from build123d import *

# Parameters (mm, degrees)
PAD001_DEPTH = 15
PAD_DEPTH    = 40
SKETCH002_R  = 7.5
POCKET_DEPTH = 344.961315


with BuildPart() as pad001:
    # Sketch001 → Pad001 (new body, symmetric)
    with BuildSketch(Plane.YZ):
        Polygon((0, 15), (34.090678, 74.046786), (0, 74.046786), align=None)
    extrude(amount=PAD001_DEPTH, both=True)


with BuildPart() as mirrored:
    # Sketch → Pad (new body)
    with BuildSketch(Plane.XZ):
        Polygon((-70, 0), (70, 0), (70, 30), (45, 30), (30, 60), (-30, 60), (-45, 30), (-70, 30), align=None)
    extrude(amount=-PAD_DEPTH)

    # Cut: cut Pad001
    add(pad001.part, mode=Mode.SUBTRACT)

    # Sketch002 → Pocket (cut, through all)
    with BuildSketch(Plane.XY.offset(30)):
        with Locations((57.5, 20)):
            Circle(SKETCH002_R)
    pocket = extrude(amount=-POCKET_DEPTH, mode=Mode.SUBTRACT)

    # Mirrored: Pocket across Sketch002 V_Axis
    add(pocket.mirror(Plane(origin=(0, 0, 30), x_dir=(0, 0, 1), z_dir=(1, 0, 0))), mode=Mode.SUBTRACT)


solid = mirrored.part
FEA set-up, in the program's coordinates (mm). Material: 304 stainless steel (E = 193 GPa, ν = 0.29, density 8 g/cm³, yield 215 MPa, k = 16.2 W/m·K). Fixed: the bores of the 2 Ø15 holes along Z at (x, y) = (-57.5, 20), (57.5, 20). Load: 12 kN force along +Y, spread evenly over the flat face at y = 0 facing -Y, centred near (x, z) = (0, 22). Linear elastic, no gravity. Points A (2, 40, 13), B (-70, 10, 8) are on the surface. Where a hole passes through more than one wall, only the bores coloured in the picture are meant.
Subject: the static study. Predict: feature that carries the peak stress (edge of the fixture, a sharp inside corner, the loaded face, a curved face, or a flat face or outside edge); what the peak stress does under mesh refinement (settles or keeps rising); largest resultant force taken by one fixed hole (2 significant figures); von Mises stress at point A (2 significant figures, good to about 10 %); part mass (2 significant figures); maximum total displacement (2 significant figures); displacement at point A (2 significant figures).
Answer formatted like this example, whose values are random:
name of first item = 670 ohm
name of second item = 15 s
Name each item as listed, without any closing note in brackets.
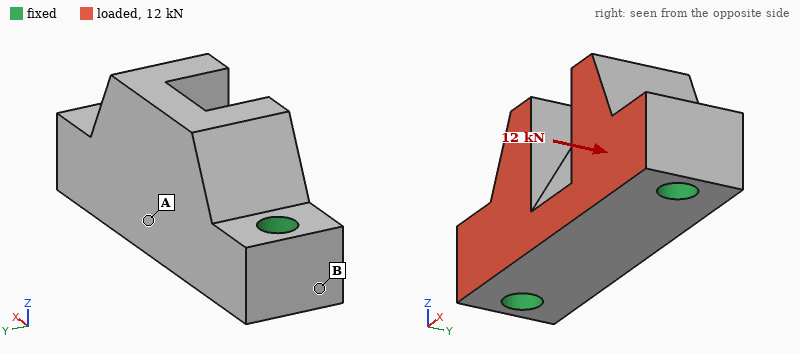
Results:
feature that carries the peak stress = edge of the fixture
what the peak stress does under mesh refinement = keeps rising
largest resultant force taken by one fixed hole = 6.0 kN
von Mises stress at point A = 6.8 MPa
part mass = 1.8 kg
maximum total displacement = 6.1 µm
displacement at point A = 3.1 µm
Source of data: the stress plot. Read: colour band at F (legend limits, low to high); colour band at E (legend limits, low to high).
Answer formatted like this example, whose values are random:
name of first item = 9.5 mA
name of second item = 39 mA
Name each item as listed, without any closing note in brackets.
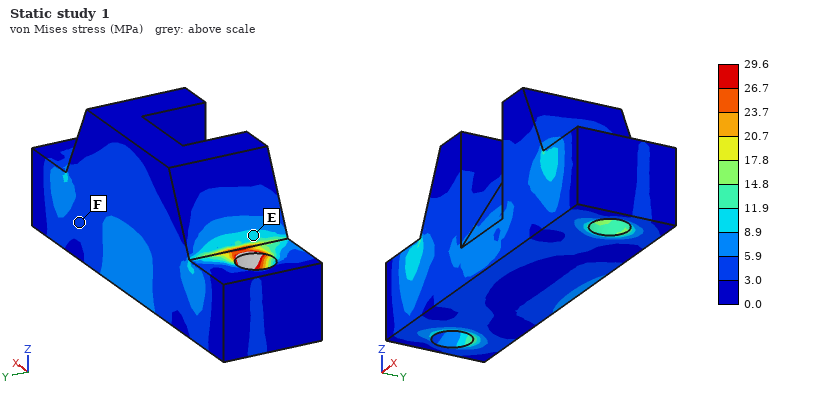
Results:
colour band at F = 3.0 to 5.9 MPa
colour band at E = 8.9 to 11.9 MPa
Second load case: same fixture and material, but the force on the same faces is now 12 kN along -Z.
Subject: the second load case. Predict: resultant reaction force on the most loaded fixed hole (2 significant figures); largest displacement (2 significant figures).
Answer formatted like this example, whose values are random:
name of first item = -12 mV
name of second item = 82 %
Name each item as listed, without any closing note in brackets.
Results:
resultant reaction force on the most loaded fixed hole = 6.1 kN
largest displacement = 8.2 µm
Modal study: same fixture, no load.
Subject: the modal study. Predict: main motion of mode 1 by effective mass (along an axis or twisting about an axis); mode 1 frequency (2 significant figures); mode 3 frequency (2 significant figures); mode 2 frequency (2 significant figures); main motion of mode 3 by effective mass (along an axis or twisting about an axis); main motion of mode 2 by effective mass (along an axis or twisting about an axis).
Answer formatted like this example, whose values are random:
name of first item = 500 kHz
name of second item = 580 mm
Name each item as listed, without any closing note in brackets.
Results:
main motion of mode 1 by effective mass = along Y
mode 1 frequency = 5700 Hz
mode 3 frequency = 9500 Hz
mode 2 frequency = 8700 Hz
main motion of mode 3 by effective mass = along Y
main motion of mode 2 by effective mass = along Z
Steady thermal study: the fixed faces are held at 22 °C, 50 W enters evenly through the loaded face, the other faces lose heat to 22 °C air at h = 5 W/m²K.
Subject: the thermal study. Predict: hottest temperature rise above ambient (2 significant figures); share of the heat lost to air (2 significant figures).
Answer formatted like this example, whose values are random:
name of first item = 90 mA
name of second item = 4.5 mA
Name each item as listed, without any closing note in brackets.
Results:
hottest temperature rise above ambient = 34 K
share of the heat lost to air = 3.6 %
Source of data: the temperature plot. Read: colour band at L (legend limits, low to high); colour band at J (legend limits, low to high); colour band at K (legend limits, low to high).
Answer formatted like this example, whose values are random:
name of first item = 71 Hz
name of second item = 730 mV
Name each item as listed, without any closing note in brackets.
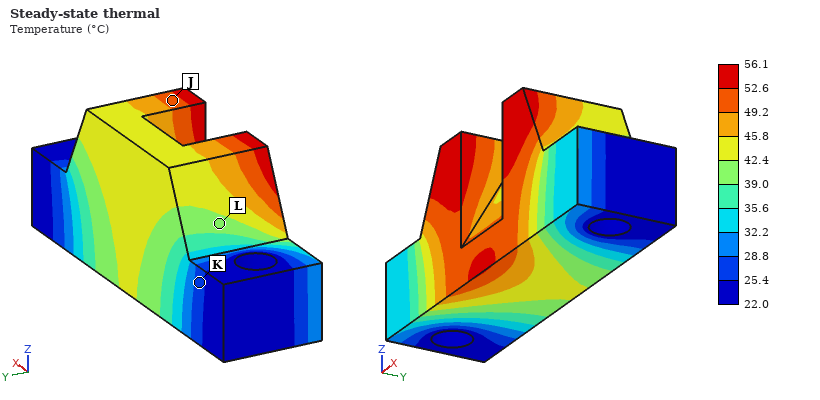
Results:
colour band at L = 39.0 to 42.4 °C
colour band at J = 49.2 to 52.6 °C
colour band at K = 25.4 to 28.8 °C
